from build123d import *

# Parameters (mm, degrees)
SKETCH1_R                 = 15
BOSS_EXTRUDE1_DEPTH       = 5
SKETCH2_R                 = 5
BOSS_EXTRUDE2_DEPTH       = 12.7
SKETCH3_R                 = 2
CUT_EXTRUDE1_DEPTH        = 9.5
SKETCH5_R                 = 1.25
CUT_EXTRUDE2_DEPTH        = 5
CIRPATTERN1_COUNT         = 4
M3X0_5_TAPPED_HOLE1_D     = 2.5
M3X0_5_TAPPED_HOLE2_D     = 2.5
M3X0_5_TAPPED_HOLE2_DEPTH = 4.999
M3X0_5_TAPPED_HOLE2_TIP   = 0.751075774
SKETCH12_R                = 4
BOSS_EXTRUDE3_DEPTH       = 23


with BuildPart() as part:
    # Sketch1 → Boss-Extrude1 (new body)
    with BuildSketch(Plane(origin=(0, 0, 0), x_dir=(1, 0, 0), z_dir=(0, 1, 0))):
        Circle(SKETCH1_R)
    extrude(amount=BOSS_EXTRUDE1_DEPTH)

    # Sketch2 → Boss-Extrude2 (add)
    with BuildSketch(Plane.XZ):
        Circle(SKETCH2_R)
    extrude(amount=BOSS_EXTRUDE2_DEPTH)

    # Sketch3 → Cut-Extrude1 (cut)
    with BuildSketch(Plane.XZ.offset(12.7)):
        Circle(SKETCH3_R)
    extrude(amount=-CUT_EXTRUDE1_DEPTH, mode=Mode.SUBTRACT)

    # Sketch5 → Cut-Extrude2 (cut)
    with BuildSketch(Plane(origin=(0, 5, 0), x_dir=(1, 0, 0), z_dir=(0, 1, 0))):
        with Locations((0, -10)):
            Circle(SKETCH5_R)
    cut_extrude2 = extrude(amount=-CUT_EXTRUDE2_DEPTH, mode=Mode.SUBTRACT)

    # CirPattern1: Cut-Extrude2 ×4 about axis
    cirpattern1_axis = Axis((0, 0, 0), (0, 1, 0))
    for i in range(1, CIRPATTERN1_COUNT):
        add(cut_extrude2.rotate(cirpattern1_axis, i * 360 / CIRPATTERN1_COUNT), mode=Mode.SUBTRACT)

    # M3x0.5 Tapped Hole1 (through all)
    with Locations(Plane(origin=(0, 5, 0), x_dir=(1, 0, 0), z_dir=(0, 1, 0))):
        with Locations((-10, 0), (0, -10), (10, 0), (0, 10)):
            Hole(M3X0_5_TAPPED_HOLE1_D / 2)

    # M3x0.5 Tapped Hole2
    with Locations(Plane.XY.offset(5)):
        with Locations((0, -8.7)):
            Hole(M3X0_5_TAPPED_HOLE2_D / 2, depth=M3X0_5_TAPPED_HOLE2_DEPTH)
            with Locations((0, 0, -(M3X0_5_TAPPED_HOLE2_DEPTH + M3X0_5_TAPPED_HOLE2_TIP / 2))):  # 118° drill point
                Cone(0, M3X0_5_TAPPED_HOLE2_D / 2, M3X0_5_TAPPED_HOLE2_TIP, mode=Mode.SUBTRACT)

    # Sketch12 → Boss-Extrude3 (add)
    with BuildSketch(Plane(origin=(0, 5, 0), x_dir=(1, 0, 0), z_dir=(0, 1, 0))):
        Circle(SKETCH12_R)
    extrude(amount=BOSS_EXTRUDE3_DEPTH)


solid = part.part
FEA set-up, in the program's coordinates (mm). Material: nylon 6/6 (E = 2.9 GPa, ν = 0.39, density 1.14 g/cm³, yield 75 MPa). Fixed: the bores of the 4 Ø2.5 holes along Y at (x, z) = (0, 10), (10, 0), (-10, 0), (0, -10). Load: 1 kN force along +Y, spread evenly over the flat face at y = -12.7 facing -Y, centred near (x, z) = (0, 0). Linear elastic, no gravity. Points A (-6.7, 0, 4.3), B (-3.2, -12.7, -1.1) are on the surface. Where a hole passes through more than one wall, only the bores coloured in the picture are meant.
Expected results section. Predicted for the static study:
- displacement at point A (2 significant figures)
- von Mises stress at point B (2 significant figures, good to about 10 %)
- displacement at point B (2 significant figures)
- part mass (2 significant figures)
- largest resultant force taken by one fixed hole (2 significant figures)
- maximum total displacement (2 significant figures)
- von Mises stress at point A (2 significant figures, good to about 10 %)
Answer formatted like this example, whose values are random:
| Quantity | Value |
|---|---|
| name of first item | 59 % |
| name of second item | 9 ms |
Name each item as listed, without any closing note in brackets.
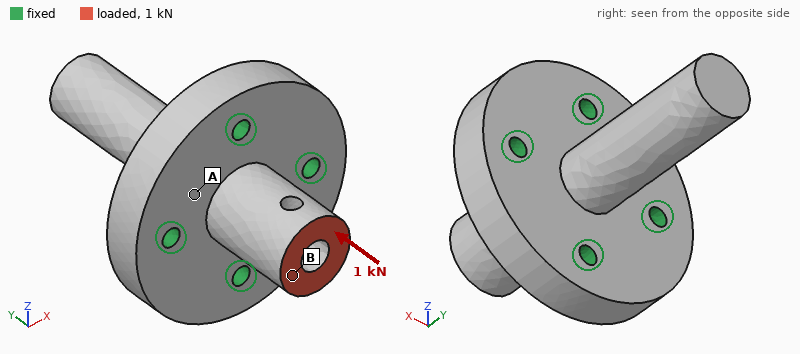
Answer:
| Quantity | Value |
|---|---|
| displacement at point A | 0.024 mm |
| von Mises stress at point B | 16 MPa |
| displacement at point B | 0.12 mm |
| part mass | 6.2 g |
| largest resultant force taken by one fixed hole | 260 N |
| maximum total displacement | 0.14 mm |
| von Mises stress at point A | 5.1 MPa |
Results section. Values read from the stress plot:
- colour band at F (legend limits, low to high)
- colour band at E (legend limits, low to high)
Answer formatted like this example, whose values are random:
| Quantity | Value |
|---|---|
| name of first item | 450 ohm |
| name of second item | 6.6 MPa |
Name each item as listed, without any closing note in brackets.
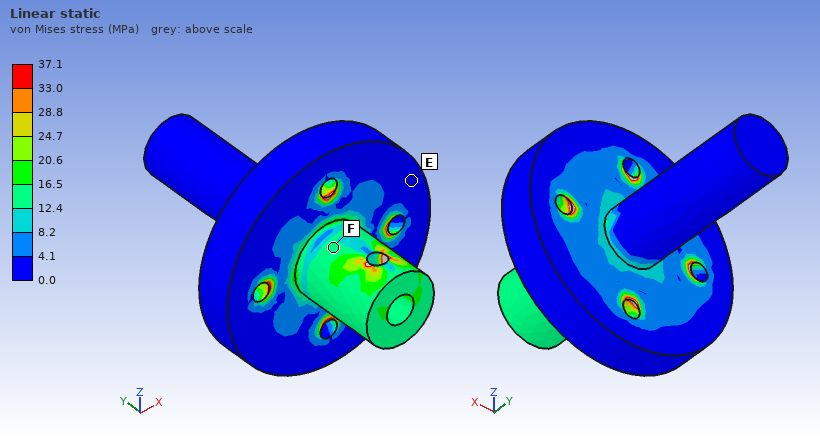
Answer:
| Quantity | Value |
|---|---|
| colour band at F | 12.4 to 16.5 MPa |
| colour band at E | 0.0 to 4.1 MPa |
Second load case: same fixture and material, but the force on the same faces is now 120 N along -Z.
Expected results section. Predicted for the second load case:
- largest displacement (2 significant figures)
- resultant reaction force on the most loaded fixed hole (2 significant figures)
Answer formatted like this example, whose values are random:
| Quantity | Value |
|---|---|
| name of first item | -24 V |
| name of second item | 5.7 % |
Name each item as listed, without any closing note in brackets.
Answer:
| Quantity | Value |
|---|---|
| largest displacement | 0.16 mm |
| resultant reaction force on the most loaded fixed hole | 100 N |
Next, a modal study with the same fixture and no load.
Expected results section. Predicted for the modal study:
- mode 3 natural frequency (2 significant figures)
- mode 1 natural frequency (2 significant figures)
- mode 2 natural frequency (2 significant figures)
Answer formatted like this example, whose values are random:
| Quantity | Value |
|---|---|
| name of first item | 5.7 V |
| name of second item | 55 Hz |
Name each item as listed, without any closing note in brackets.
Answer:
| Quantity | Value |
|---|---|
| mode 3 natural frequency | 8300 Hz |
| mode 1 natural frequency | 2700 Hz |
| mode 2 natural frequency | 2700 Hz |
